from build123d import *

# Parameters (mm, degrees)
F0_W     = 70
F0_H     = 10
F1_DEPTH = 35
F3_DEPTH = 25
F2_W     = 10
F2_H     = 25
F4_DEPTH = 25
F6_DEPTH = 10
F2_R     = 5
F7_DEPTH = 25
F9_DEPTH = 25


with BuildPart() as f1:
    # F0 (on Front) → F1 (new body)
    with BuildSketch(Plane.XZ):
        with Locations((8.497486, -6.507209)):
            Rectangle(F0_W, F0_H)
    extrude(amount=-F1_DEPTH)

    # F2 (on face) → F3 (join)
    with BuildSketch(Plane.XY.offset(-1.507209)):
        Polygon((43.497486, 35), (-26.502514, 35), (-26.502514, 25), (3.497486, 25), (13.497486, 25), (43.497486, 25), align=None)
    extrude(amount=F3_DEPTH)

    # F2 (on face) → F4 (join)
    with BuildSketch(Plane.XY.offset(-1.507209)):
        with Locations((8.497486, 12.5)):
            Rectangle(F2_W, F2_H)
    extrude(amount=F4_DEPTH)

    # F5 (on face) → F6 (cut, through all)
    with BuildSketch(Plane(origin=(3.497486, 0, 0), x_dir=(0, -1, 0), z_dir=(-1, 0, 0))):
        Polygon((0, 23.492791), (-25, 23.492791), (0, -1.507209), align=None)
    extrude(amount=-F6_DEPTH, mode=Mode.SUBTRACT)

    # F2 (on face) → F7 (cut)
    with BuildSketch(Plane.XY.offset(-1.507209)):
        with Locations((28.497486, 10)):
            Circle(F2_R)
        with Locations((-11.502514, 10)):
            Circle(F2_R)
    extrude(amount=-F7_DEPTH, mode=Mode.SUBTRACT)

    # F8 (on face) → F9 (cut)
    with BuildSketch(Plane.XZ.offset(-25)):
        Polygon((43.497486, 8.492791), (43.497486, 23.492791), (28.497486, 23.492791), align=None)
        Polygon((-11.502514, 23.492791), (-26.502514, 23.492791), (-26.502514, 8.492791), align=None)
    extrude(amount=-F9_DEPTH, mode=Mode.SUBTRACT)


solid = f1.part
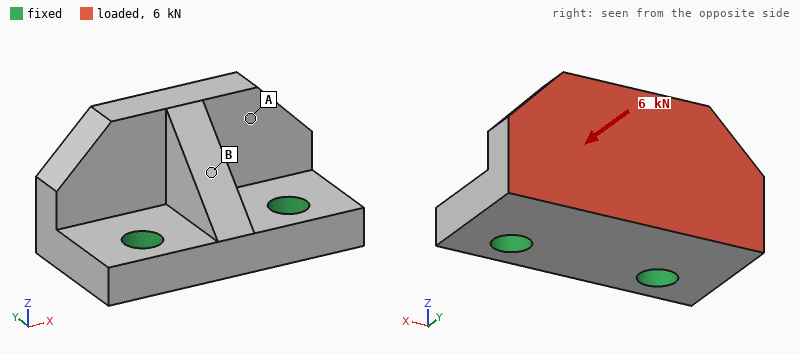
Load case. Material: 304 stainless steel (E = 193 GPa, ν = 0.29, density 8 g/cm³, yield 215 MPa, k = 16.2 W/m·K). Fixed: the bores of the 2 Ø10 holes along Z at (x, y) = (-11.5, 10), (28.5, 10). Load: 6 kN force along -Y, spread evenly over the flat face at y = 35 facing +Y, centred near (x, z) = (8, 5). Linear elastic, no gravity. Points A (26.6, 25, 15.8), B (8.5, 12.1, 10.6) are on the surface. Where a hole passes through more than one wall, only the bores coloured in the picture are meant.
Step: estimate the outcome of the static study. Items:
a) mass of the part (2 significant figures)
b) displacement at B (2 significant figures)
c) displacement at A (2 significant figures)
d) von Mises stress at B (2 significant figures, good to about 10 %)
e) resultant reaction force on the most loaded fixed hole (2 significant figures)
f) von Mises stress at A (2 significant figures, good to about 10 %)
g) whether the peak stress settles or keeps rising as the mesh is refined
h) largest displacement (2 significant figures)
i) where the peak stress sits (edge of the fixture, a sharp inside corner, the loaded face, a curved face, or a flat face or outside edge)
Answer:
330 g
11 µm
17 µm
26 MPa
3.0 kN
9.3 MPa
keeps rising
25 µm
edge of the fixture
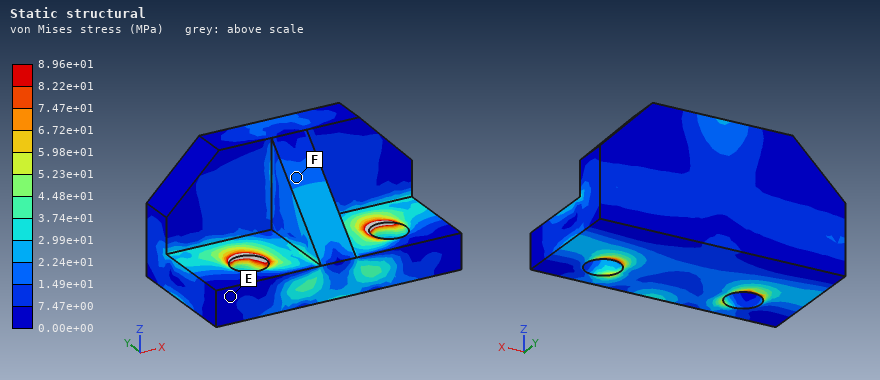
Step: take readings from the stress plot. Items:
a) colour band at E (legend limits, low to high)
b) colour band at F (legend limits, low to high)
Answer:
0.00e+00 to 7.47e+00 MPa
1.49e+01 to 2.24e+01 MPa
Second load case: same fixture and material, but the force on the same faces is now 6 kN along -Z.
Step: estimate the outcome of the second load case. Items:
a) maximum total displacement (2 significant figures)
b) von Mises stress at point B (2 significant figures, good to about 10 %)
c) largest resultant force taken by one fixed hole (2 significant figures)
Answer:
39 µm
27 MPa
3.0 kN
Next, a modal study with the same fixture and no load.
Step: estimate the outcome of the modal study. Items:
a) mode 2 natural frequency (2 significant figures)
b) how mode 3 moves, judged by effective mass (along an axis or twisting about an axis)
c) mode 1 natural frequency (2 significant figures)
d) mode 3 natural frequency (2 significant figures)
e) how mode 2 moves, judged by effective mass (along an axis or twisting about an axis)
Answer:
9000 Hz
along X
5700 Hz
14 kHz
along X
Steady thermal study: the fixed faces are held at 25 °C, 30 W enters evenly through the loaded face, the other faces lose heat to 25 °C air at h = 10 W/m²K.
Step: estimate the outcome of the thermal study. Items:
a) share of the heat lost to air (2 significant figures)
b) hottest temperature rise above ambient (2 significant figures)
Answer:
8.3 %
64 K
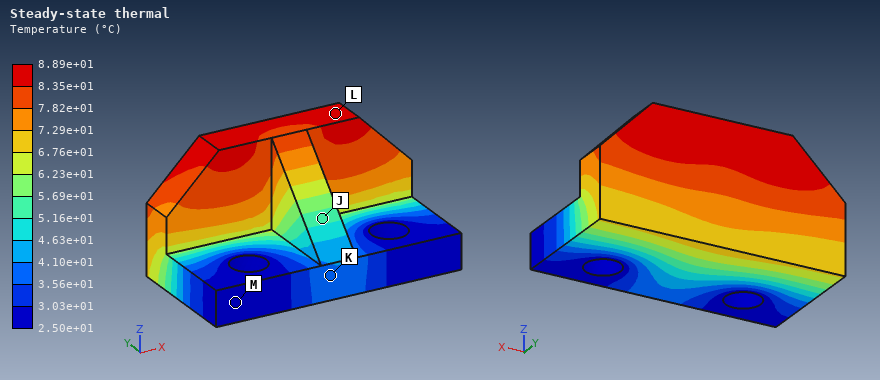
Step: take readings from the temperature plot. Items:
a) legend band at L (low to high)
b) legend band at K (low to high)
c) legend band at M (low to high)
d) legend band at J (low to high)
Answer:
8.35e+01 to 8.89e+01 °C
3.56e+01 to 4.10e+01 °C
2.50e+01 to 3.03e+01 °C
5.16e+01 to 5.69e+01 °C
